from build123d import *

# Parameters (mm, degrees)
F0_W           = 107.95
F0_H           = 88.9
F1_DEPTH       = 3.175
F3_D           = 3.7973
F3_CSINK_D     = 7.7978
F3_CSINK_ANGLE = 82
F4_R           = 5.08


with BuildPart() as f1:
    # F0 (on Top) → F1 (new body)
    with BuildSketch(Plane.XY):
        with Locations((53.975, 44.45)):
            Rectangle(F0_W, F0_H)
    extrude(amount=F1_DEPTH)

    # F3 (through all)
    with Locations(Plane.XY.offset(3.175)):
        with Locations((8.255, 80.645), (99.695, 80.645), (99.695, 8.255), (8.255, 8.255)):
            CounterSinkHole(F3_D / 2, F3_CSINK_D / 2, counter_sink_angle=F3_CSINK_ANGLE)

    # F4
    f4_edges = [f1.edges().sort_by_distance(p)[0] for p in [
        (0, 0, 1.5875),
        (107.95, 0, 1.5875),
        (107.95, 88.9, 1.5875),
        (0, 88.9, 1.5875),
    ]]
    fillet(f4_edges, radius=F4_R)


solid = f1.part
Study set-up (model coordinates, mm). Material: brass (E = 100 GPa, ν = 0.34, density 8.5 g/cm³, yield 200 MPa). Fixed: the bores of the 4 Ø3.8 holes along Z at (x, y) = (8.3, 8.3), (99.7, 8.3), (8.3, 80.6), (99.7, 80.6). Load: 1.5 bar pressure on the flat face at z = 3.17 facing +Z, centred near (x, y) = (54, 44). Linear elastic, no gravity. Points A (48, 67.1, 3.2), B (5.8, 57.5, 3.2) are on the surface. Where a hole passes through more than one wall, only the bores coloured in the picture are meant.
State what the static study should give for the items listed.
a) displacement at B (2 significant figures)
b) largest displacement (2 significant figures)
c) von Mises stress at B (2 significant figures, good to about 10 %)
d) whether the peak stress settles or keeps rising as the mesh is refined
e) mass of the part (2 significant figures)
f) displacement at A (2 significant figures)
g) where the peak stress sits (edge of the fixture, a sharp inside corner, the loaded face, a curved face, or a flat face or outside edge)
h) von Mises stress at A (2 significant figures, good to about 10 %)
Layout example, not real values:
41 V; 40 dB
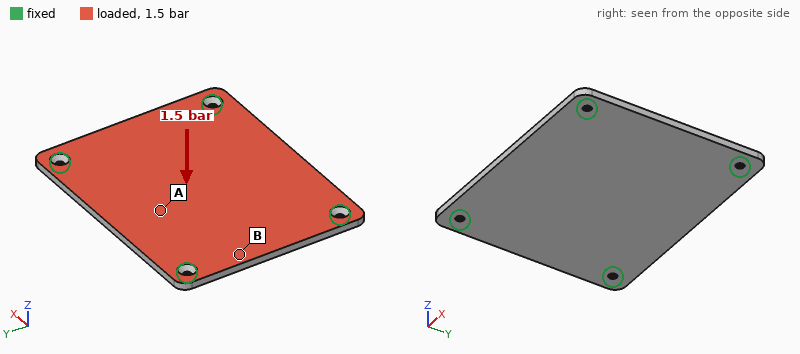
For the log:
0.063 mm; 0.26 mm; 28 MPa; keeps rising; 260 g; 0.23 mm; edge of the fixture; 47 MPa
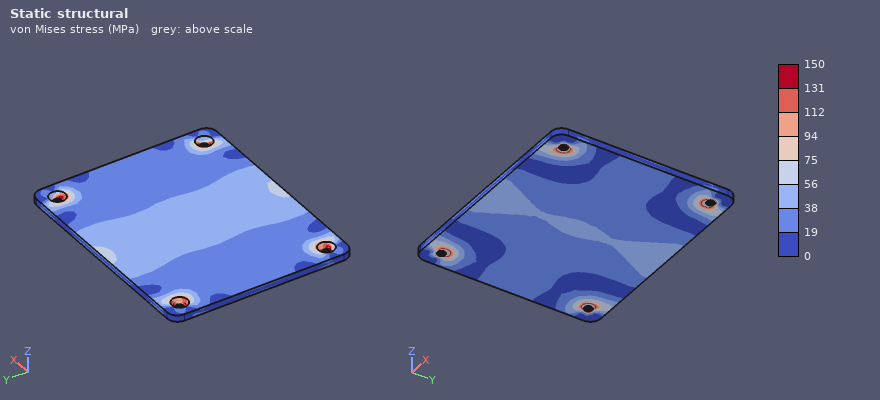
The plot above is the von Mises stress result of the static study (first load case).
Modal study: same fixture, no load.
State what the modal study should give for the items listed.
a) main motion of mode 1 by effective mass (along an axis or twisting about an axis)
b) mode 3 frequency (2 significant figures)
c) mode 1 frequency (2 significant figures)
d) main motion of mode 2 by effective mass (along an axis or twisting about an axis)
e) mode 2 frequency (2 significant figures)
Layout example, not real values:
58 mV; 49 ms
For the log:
along Z; 1700 Hz; 870 Hz; twisting about X; 1400 Hz
